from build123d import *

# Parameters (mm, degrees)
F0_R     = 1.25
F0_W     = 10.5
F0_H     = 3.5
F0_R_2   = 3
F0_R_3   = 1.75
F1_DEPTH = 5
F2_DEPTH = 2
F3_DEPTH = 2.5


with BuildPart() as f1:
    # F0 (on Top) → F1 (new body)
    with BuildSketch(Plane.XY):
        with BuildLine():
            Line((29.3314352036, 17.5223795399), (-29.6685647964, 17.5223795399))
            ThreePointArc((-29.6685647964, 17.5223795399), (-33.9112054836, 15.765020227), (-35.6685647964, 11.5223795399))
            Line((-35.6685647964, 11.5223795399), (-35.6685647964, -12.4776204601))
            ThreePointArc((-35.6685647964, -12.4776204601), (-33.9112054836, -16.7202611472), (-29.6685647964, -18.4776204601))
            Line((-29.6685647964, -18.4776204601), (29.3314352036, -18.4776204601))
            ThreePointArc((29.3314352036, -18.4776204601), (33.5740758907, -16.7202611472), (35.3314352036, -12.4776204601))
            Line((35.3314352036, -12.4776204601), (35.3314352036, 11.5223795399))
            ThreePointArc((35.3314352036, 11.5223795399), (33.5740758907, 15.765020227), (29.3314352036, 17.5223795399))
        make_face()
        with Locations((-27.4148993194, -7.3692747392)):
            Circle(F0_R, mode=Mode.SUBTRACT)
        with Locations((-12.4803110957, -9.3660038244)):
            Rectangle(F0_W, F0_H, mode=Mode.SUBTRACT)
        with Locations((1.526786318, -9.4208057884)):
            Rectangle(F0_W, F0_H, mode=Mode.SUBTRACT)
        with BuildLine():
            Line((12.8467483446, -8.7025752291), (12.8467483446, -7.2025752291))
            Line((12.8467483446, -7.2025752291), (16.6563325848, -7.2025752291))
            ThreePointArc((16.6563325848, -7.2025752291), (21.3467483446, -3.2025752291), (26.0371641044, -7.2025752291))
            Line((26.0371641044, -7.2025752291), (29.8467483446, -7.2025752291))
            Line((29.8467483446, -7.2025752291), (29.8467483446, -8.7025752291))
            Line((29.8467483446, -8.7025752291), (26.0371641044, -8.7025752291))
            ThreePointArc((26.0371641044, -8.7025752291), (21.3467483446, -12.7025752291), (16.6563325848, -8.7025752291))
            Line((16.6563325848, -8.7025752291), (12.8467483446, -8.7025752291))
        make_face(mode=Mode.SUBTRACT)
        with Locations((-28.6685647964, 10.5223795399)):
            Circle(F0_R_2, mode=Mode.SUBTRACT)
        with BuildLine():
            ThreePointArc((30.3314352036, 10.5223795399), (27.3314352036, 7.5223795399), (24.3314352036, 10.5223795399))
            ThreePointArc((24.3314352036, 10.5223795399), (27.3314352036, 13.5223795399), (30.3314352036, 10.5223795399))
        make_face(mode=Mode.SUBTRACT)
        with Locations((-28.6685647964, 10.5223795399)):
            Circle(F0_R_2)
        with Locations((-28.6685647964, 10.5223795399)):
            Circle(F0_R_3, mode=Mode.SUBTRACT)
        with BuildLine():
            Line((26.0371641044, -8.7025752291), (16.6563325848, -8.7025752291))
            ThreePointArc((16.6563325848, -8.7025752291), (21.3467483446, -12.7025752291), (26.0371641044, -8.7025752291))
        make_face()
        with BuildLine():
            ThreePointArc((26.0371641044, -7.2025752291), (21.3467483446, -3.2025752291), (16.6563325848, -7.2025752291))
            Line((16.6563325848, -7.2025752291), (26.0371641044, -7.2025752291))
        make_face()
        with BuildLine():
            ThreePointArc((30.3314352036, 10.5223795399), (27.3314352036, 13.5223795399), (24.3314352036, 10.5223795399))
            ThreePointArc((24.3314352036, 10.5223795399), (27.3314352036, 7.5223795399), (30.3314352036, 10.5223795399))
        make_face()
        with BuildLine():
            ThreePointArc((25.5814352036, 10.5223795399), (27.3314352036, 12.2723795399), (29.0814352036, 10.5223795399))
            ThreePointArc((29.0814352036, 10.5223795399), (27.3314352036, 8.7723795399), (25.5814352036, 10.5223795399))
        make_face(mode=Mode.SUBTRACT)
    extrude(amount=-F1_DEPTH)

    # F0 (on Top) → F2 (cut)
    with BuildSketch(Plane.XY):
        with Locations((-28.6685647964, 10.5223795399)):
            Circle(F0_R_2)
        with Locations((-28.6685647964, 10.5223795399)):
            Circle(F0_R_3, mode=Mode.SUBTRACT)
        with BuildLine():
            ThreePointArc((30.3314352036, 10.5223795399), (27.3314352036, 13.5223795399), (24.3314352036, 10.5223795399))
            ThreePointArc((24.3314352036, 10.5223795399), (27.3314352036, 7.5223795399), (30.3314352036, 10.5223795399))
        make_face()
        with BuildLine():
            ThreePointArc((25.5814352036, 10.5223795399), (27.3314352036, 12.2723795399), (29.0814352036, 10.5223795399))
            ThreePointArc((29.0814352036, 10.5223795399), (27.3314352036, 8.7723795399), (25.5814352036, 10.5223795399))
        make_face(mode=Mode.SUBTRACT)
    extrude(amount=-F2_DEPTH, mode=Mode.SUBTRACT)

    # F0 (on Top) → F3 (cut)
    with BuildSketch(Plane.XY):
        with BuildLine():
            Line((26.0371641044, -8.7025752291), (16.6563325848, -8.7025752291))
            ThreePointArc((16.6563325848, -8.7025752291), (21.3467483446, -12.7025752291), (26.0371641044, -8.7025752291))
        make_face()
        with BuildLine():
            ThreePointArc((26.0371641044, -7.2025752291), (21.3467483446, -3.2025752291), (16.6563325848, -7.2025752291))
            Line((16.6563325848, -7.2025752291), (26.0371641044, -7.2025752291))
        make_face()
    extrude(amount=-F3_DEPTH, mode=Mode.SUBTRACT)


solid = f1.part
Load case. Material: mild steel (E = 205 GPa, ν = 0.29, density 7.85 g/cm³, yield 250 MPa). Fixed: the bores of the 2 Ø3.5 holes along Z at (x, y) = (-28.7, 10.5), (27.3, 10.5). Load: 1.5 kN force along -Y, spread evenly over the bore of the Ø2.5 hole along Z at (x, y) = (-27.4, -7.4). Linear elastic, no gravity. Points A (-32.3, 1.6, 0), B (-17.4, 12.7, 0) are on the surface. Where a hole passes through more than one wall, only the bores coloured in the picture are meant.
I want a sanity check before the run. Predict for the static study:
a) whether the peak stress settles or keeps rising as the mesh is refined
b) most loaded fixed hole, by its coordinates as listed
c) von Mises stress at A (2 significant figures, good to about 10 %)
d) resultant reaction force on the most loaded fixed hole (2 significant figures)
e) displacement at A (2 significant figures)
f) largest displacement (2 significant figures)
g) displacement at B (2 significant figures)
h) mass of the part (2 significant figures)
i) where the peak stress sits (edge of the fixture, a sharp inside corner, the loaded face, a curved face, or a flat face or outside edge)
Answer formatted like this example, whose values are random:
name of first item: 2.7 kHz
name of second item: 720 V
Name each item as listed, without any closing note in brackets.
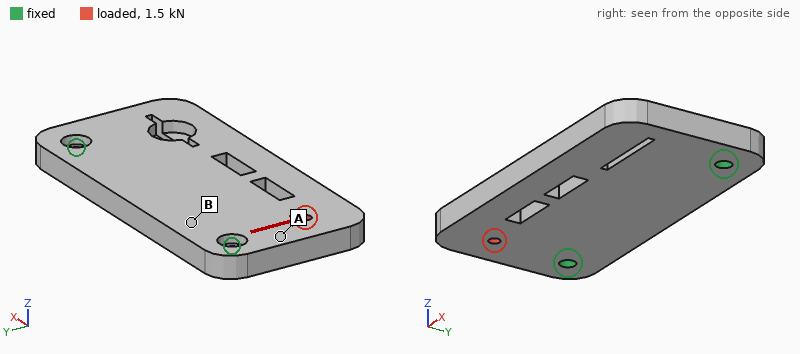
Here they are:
whether the peak stress settles or keeps rising as the mesh is refined: keeps rising
most loaded fixed hole, by its coordinates as listed: (-28.7, 10.5)
von Mises stress at A: 17 MPa
resultant reaction force on the most loaded fixed hole: 1.5 kN
displacement at A: 3.1 µm
largest displacement: 7.2 µm
displacement at B: 1.7 µm
mass of the part: 93 g
where the peak stress sits: edge of the fixture
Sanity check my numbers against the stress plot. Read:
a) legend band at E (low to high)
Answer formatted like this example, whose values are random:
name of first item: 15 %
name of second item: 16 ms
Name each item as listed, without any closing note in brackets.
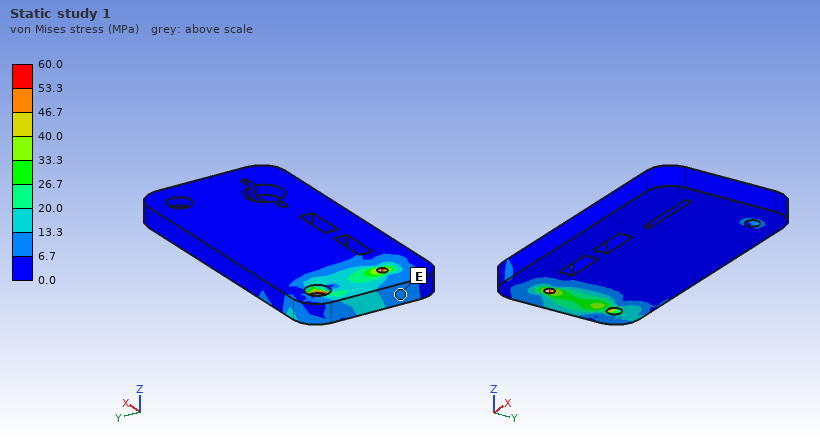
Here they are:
legend band at E: 6.7 to 13.3 MPa
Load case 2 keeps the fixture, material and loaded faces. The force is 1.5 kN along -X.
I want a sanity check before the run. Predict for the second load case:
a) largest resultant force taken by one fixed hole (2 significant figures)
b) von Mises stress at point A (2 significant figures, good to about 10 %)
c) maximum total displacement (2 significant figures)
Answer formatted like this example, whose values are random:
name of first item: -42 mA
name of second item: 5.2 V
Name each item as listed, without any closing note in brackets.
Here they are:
largest resultant force taken by one fixed hole: 930 N
von Mises stress at point A: 6.1 MPa
maximum total displacement: 4.2 µm
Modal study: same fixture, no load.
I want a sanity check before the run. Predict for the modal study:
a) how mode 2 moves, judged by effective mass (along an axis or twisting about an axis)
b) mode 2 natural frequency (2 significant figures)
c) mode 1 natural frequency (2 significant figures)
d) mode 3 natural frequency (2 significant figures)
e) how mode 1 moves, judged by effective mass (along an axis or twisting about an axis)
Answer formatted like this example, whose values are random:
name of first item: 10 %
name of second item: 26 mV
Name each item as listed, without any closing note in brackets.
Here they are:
how mode 2 moves, judged by effective mass: twisting about Y
mode 2 natural frequency: 5400 Hz
mode 1 natural frequency: 2700 Hz
mode 3 natural frequency: 6600 Hz
how mode 1 moves, judged by effective mass: along Z
